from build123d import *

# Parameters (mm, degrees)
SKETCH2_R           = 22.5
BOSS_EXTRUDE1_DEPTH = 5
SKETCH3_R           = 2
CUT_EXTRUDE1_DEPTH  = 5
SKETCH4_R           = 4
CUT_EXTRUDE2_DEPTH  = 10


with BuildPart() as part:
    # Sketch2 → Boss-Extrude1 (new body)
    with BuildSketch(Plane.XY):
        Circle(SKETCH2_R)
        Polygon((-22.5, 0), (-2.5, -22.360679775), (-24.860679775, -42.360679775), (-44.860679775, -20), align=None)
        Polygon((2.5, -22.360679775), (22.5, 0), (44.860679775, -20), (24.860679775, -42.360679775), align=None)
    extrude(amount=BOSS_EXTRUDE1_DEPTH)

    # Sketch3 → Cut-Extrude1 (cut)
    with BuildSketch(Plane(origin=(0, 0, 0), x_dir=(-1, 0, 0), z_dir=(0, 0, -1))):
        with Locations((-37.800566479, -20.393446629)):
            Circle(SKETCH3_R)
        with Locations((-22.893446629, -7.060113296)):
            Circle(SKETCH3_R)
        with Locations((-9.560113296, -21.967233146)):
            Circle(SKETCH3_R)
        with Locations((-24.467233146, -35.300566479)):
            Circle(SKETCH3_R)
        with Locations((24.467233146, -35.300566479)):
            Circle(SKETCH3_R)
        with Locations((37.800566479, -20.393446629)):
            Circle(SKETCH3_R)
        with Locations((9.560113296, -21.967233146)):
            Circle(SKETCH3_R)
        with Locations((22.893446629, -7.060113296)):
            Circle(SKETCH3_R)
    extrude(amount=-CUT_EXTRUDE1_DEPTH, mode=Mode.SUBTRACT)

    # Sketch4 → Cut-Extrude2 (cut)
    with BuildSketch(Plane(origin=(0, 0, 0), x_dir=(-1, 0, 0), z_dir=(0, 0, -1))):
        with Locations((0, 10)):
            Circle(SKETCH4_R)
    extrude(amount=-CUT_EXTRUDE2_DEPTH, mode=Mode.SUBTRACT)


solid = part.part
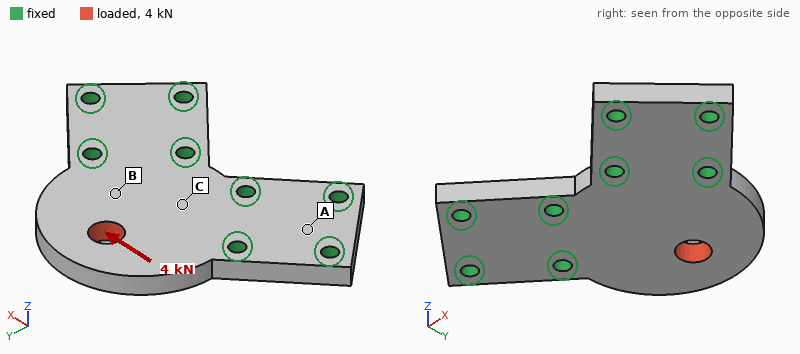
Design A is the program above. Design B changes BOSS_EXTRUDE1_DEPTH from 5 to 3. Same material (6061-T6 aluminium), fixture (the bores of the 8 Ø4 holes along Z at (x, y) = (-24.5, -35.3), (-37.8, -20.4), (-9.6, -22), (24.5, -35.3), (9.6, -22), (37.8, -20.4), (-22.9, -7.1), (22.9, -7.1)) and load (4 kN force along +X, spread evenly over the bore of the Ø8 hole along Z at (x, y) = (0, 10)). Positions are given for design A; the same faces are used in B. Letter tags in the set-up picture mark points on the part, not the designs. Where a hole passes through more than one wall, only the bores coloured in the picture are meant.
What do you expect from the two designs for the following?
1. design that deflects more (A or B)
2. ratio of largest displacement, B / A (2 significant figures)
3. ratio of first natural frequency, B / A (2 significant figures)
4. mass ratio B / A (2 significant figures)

B
1.7
0.63
0.60
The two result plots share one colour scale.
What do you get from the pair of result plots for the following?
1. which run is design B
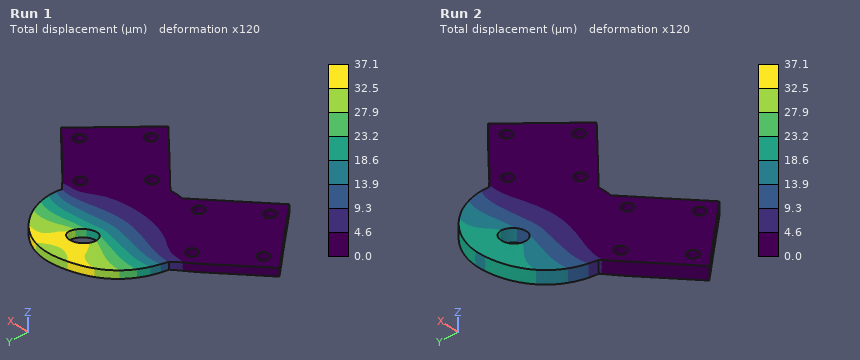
Run 1
